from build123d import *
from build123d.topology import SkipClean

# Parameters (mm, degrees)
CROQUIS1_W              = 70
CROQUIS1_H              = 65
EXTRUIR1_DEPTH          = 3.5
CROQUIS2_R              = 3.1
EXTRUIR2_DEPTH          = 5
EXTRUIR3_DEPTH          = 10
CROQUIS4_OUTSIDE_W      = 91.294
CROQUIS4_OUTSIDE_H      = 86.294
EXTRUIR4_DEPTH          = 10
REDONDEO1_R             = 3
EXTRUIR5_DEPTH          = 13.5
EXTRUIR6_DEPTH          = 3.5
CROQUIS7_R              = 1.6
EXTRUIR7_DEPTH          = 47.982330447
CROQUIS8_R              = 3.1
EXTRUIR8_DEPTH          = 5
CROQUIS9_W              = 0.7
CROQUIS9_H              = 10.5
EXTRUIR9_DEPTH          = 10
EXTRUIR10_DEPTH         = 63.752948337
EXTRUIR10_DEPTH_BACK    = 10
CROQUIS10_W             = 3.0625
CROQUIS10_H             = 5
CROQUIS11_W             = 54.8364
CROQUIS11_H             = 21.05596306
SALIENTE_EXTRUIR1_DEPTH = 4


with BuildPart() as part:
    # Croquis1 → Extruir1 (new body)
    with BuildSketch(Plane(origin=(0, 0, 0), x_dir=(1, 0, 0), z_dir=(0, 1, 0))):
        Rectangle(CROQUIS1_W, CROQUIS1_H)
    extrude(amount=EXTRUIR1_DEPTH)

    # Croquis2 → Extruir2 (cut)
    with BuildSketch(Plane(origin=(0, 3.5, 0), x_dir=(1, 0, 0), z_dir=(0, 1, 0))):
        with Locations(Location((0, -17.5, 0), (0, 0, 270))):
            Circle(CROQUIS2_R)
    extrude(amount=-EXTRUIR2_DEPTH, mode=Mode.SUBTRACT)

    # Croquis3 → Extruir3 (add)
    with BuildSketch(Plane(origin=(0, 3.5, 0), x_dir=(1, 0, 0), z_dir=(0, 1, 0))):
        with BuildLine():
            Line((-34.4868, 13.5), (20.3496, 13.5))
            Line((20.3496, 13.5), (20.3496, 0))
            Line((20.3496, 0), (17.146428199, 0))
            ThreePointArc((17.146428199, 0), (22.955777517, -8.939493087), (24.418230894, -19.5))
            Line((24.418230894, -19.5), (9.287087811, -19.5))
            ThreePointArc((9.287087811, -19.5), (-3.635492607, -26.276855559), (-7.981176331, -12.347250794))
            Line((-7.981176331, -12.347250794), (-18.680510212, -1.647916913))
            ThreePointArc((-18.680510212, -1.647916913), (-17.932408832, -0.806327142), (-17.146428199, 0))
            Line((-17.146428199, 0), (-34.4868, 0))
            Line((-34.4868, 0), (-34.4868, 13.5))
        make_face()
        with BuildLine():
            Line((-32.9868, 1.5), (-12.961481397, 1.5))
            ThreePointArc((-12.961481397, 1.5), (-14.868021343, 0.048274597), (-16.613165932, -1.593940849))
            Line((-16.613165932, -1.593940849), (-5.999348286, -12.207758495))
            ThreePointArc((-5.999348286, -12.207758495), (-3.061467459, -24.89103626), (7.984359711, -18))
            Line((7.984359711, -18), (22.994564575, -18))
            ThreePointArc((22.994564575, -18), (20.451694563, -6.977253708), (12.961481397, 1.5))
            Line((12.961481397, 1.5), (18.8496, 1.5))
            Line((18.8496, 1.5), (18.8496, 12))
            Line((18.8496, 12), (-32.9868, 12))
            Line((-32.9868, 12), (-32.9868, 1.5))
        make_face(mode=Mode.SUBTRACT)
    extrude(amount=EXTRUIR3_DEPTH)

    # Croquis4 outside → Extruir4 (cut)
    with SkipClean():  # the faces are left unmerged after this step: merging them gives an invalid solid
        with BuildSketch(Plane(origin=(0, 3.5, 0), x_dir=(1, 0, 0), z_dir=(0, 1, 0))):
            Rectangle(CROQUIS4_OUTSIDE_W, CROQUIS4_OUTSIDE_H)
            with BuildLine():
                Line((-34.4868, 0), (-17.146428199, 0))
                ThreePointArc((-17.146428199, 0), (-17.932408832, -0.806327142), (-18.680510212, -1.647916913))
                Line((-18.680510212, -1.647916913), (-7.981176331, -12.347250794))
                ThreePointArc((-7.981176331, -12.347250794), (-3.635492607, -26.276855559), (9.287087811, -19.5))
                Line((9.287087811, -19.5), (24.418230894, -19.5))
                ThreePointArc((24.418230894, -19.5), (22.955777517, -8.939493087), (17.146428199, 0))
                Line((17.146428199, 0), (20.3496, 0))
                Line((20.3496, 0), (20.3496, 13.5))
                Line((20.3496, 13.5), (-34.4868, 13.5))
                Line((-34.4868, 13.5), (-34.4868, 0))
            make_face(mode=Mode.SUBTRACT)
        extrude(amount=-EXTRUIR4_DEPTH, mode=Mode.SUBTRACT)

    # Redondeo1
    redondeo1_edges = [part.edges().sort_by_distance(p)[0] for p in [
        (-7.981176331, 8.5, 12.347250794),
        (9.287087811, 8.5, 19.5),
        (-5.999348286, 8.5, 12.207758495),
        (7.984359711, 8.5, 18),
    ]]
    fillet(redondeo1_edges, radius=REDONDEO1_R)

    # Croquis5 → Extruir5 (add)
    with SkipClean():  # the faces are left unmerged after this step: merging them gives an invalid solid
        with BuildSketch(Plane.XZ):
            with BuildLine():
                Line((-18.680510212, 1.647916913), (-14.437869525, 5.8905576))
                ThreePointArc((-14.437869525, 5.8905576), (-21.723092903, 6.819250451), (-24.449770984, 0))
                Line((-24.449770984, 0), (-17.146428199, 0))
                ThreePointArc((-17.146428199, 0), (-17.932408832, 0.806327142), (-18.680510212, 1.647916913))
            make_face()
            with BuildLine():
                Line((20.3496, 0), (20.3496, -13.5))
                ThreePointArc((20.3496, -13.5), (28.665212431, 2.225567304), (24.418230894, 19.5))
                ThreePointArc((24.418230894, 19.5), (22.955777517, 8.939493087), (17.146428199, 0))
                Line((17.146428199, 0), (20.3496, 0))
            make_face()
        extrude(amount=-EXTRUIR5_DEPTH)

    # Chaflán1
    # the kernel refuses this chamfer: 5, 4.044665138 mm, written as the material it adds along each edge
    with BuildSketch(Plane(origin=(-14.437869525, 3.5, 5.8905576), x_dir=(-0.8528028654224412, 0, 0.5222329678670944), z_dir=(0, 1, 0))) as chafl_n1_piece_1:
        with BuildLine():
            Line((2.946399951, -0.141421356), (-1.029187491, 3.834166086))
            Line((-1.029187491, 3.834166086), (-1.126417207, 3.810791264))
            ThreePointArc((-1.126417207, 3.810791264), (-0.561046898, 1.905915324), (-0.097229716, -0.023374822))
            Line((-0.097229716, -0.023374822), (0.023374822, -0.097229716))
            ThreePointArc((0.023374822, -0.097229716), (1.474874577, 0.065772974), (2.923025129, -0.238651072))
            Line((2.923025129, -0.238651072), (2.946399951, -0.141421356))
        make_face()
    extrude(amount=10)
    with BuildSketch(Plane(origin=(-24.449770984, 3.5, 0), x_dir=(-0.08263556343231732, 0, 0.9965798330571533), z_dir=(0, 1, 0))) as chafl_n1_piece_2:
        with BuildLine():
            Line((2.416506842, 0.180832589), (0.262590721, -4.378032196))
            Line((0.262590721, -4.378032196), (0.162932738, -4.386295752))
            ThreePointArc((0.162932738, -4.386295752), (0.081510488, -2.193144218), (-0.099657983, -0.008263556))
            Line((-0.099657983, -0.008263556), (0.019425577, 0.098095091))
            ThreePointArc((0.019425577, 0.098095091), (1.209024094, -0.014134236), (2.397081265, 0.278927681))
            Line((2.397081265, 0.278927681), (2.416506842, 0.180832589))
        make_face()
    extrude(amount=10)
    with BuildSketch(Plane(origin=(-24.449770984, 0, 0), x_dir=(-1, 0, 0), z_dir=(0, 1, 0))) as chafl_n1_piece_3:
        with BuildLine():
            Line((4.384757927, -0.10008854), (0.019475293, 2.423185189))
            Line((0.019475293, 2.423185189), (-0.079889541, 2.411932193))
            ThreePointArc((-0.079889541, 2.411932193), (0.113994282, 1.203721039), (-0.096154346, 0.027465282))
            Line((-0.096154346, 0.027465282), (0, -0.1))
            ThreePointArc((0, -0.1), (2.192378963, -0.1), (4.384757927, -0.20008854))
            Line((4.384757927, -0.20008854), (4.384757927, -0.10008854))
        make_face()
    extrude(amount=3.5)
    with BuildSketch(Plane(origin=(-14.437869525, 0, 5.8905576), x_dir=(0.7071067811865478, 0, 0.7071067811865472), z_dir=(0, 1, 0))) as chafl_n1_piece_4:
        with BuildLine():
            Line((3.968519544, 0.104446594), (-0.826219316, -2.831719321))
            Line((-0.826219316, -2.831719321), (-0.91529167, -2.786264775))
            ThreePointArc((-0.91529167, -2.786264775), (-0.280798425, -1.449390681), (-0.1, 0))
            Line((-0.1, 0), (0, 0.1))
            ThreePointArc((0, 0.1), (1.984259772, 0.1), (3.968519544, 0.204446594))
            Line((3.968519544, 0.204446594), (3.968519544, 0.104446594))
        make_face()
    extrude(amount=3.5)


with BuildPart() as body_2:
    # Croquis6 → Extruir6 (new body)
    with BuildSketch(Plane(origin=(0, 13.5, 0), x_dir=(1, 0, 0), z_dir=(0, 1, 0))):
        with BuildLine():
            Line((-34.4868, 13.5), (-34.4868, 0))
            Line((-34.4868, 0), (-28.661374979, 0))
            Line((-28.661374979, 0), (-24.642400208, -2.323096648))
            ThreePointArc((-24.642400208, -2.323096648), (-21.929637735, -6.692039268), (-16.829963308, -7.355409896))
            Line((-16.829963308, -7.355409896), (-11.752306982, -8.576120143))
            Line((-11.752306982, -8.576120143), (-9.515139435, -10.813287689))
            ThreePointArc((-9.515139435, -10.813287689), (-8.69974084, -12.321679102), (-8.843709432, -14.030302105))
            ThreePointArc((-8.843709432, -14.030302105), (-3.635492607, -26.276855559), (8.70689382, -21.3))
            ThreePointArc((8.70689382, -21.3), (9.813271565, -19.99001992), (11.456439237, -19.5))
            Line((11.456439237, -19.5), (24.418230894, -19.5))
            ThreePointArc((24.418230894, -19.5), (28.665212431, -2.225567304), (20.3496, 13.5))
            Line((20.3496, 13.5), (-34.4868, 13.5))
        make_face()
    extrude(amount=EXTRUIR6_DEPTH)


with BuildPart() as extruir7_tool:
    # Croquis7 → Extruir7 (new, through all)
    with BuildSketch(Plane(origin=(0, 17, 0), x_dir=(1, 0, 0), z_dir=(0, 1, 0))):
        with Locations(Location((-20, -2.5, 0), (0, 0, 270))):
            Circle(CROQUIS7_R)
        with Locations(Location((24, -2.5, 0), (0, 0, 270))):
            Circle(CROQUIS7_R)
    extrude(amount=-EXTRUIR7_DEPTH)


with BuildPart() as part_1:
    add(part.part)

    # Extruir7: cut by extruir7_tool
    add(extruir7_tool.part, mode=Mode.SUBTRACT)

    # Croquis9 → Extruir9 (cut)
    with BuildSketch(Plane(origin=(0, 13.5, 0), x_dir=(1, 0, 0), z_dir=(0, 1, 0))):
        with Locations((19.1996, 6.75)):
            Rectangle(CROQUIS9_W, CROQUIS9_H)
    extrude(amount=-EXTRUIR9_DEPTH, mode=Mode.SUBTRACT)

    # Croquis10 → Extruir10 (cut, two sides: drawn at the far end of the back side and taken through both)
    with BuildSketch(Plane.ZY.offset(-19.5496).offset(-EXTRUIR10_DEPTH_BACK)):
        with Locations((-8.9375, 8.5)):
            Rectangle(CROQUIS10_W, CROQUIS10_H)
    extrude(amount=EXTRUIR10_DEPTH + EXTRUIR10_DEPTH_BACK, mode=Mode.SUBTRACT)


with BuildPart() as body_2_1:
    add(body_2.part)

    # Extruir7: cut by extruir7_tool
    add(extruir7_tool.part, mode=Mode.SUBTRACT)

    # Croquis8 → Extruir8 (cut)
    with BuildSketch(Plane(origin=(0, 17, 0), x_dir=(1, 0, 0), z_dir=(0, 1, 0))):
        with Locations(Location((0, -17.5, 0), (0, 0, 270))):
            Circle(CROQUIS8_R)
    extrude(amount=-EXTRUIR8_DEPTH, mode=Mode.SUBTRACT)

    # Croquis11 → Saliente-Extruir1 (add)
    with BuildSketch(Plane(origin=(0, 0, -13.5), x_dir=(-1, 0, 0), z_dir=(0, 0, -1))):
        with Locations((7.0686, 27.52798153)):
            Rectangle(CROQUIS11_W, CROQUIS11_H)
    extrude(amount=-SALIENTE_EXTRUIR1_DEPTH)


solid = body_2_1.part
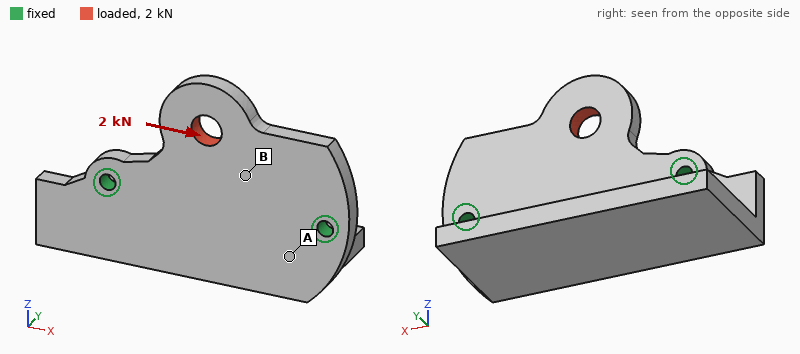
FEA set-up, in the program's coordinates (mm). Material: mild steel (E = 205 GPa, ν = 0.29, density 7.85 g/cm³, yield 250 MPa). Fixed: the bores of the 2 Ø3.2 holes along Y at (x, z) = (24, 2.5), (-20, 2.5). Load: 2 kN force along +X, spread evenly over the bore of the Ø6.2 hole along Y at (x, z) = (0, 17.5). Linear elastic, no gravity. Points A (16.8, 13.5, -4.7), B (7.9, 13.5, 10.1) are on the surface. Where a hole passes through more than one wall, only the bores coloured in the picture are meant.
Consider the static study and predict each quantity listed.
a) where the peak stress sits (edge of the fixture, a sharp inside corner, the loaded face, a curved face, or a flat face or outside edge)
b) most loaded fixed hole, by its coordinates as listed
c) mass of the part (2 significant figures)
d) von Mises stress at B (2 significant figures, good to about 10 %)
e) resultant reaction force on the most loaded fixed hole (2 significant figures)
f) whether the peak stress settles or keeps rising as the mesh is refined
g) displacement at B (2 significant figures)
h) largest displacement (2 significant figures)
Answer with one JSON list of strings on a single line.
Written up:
["edge of the fixture", "(24, 2.5)", "83 g", "21 MPa", "1.4 kN", "keeps rising", "2.8 µm", "8.5 µm"]
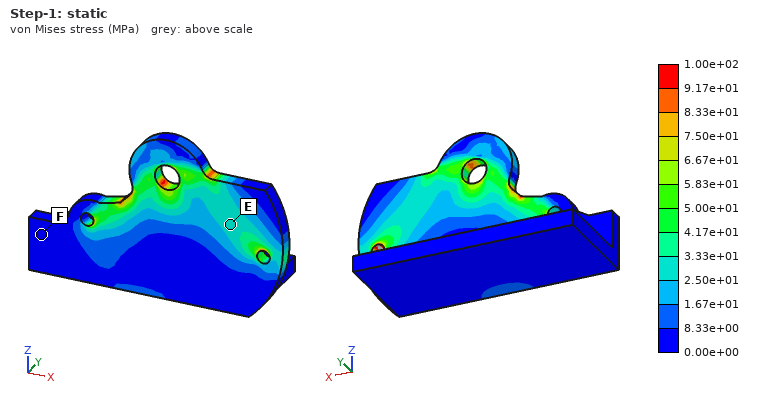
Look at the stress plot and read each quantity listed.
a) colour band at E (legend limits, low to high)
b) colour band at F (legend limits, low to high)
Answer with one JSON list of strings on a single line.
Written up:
["2.50e+01 to 3.33e+01 MPa", "0.00e+00 to 8.33e+00 MPa"]
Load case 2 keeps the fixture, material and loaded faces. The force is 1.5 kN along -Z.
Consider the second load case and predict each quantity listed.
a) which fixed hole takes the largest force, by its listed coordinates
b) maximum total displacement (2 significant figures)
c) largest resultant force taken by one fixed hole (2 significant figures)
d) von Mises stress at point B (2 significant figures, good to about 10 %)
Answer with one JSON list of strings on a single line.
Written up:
["(-20, 2.5)", "5.3 µm", "820 N", "13 MPa"]
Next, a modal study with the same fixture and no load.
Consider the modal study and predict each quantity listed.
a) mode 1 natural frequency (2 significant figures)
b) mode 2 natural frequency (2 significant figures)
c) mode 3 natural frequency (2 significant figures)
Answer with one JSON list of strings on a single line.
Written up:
["2200 Hz", "4500 Hz", "4900 Hz"]
